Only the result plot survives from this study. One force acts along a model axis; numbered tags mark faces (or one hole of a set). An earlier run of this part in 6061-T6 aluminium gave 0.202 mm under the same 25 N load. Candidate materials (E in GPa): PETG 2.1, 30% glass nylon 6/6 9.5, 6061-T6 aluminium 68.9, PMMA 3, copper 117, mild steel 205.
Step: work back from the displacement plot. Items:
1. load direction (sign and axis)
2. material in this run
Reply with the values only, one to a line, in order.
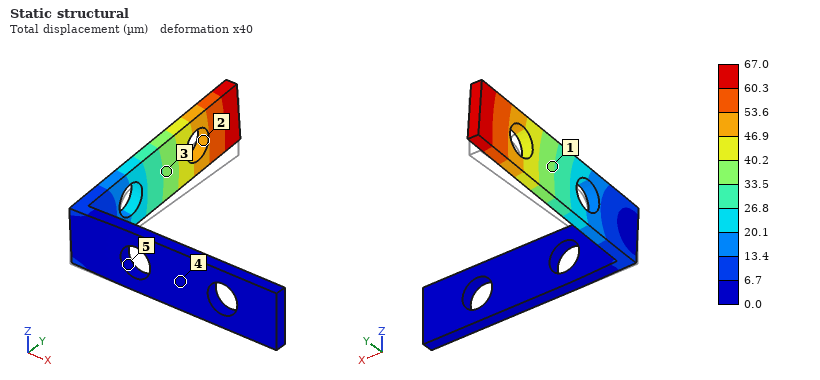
+Z
mild steel
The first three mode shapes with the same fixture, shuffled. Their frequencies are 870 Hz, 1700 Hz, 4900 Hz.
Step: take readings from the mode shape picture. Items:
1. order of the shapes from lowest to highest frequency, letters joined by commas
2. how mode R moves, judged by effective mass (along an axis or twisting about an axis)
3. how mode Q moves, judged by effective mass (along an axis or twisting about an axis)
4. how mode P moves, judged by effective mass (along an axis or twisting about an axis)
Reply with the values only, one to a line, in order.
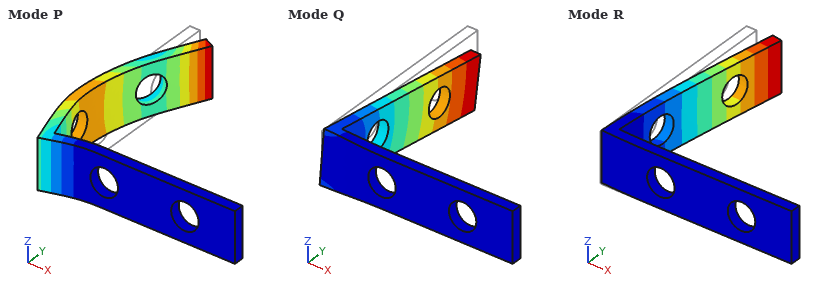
R, Q, P
along X
along Z
along Y
